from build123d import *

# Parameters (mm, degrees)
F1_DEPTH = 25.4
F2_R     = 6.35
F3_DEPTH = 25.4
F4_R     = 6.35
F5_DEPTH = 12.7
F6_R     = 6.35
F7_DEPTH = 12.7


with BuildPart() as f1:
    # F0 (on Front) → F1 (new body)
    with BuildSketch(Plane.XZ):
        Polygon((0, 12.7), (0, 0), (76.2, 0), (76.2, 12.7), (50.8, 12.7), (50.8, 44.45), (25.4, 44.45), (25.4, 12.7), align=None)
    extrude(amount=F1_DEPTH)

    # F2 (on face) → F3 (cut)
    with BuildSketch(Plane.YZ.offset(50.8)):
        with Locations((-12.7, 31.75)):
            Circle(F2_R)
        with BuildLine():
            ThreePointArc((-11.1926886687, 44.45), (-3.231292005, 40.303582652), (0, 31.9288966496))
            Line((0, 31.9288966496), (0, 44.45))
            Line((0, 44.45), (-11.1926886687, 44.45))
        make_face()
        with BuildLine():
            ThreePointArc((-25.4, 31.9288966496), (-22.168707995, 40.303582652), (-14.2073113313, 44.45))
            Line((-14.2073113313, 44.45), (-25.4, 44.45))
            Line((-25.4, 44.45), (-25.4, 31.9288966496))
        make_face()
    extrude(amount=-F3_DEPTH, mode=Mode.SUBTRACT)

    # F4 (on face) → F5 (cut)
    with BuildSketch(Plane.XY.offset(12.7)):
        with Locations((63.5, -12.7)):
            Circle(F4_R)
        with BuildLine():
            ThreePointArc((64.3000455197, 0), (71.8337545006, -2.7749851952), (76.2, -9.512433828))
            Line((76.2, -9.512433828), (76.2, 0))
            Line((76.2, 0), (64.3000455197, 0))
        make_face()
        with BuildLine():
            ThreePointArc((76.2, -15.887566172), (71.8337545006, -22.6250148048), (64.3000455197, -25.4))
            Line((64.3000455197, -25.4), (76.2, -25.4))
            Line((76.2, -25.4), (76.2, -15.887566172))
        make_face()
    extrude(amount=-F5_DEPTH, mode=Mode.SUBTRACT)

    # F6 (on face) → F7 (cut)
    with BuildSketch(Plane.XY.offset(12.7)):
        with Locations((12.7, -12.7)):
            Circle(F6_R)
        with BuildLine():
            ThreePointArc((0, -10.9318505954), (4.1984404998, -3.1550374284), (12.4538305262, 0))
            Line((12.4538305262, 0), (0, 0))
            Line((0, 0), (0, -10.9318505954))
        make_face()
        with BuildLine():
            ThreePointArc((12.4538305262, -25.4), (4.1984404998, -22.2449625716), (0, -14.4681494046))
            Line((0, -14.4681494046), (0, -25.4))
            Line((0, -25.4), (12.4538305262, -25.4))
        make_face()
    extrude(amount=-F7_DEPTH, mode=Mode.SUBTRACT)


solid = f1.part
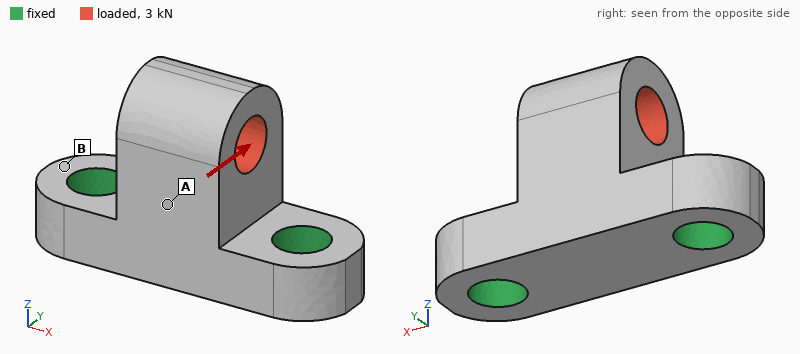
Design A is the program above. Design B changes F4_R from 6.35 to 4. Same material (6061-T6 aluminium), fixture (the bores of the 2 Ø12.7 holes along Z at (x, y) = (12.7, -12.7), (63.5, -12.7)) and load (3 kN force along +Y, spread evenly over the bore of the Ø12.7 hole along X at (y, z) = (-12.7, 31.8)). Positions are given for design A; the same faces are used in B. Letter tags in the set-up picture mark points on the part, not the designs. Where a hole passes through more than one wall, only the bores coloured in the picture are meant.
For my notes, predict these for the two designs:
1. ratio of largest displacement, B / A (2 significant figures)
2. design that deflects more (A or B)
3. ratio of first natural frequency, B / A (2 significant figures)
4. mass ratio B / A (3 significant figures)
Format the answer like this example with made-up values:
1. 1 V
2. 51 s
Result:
1. 1.1
2. B
3. 0.94
4. 1.03
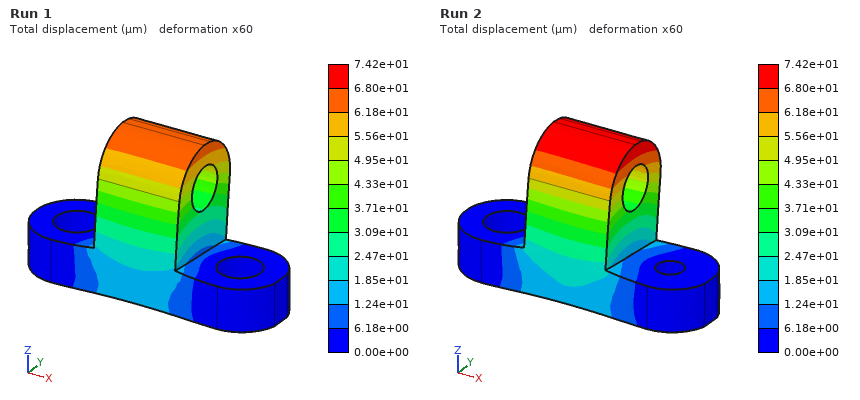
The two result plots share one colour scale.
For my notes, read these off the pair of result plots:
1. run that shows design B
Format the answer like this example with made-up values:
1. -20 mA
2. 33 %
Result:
1. Run 2
